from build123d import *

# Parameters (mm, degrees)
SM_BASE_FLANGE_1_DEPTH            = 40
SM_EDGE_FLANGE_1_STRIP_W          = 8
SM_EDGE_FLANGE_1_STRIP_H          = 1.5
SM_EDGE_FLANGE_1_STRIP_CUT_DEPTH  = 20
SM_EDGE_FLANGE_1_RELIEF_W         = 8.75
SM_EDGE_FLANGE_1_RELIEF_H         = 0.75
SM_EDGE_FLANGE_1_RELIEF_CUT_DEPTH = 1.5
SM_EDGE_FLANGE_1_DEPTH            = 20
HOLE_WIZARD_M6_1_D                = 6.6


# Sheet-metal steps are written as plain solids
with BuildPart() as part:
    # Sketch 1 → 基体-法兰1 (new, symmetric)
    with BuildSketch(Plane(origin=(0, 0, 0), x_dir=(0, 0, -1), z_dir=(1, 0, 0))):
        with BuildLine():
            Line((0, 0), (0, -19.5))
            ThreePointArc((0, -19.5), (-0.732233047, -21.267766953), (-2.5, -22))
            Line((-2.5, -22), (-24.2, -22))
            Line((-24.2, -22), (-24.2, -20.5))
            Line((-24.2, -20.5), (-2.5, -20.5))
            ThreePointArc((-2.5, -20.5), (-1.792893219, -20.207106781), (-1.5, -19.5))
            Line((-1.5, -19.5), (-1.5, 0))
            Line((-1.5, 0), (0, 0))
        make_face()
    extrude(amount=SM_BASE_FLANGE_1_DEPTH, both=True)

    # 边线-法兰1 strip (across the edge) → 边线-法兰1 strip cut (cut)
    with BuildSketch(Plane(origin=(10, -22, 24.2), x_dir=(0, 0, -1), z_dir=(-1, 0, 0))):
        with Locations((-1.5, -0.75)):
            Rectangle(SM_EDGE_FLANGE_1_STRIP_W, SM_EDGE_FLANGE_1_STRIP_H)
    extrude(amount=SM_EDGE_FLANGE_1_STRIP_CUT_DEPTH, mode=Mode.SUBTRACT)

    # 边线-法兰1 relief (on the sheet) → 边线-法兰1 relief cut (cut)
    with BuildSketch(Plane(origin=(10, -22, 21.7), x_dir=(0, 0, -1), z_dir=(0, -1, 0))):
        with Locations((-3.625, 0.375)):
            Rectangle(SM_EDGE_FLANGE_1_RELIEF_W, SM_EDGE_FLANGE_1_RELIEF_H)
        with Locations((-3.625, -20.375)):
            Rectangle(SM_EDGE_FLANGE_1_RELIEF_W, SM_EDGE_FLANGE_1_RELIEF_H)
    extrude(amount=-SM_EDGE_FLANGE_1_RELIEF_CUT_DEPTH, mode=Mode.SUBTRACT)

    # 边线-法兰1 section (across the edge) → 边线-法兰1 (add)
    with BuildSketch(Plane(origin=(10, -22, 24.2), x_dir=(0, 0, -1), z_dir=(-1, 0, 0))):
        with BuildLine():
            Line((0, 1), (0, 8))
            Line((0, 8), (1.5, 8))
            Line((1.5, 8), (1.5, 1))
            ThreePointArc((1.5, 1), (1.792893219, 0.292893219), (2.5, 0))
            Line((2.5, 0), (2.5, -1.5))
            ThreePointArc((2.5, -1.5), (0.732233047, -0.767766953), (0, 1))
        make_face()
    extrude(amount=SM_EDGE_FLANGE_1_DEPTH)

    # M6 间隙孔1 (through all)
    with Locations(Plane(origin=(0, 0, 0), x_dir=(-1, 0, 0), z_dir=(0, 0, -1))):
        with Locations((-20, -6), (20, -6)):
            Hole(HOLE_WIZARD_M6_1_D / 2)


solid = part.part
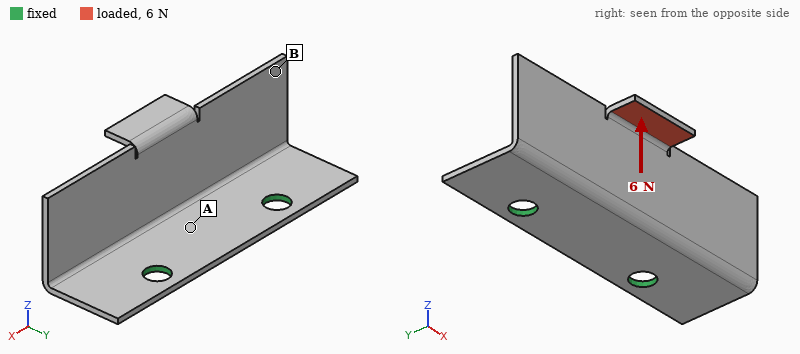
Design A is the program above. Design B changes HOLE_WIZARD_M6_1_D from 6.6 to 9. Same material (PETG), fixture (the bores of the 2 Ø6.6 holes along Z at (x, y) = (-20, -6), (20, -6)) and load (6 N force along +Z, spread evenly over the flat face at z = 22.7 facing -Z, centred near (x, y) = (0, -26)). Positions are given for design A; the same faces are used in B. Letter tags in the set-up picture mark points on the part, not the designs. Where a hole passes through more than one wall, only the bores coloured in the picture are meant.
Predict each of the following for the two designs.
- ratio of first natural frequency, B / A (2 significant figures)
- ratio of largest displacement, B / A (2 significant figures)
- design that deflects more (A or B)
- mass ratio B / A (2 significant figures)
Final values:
1.1
0.88
A
0.98
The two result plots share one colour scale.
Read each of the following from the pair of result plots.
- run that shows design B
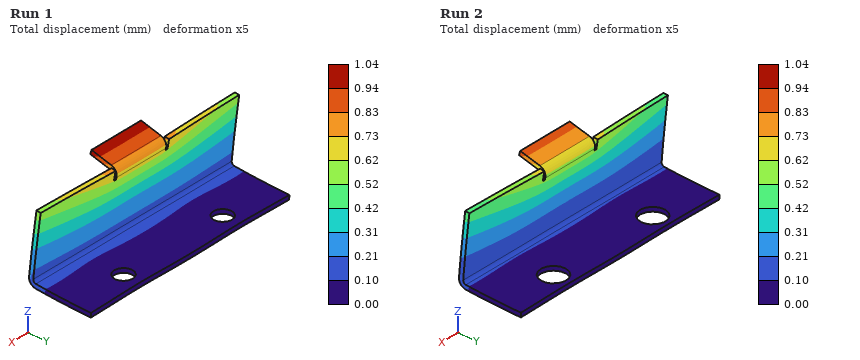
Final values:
Run 2
